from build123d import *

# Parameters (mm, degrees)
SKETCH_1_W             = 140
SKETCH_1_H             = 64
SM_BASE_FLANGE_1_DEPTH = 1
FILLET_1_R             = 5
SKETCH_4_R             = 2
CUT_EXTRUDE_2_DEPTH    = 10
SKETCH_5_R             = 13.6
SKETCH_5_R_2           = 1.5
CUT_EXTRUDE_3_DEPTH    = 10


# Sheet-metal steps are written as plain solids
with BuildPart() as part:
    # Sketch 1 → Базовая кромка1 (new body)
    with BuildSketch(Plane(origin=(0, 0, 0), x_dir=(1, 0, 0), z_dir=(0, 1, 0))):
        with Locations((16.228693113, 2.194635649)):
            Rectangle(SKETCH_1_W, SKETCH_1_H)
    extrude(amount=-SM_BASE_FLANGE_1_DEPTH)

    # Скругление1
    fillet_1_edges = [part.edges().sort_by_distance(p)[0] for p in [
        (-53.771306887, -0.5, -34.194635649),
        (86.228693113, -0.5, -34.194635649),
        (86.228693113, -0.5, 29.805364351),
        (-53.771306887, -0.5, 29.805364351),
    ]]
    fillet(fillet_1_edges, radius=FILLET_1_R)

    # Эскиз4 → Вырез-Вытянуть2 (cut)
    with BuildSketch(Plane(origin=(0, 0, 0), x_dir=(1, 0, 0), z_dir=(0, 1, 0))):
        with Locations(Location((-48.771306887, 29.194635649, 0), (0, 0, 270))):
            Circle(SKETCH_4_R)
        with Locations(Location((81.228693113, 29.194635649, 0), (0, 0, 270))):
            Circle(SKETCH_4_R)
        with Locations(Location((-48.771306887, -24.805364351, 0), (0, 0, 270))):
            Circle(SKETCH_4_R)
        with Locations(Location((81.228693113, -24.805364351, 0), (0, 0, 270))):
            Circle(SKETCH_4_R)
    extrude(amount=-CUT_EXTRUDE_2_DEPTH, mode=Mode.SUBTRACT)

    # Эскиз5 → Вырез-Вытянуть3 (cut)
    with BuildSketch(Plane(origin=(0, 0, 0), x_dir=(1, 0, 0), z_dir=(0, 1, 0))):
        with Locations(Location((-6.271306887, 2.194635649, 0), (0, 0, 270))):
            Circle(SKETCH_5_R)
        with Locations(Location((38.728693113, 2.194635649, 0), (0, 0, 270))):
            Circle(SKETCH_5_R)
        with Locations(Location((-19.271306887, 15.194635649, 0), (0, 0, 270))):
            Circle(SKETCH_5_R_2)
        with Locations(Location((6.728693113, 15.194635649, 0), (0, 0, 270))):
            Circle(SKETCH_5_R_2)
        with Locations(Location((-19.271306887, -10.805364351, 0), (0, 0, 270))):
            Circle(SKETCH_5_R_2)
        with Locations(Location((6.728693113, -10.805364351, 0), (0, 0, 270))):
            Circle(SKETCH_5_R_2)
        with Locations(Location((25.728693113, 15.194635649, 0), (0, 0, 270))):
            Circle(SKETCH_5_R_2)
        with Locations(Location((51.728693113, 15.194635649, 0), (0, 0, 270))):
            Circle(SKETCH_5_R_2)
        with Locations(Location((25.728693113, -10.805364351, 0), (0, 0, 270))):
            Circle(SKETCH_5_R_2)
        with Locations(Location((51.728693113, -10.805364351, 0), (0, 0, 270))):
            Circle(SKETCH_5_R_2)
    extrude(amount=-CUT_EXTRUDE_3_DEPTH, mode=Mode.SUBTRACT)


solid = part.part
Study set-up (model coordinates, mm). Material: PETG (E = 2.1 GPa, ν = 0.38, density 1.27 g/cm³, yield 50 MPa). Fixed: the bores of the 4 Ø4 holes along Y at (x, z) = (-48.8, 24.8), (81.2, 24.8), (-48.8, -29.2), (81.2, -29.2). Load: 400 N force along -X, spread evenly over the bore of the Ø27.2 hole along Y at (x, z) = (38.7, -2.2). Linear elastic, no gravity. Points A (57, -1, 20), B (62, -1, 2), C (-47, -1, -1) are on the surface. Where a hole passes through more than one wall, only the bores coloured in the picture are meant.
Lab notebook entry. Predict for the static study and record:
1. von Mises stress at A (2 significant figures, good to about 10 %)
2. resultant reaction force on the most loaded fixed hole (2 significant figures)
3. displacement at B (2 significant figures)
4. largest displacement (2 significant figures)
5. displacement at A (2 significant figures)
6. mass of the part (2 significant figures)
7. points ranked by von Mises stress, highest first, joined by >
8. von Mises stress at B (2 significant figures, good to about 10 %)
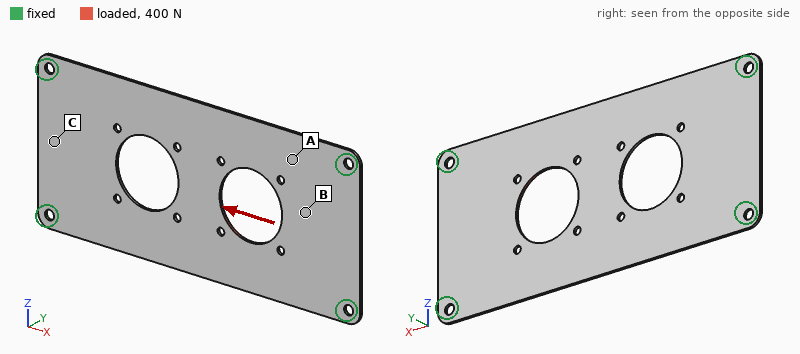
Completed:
5.4 MPa
140 N
0.12 mm
0.19 mm
0.093 mm
9.7 g
A > B > C
3.2 MPa
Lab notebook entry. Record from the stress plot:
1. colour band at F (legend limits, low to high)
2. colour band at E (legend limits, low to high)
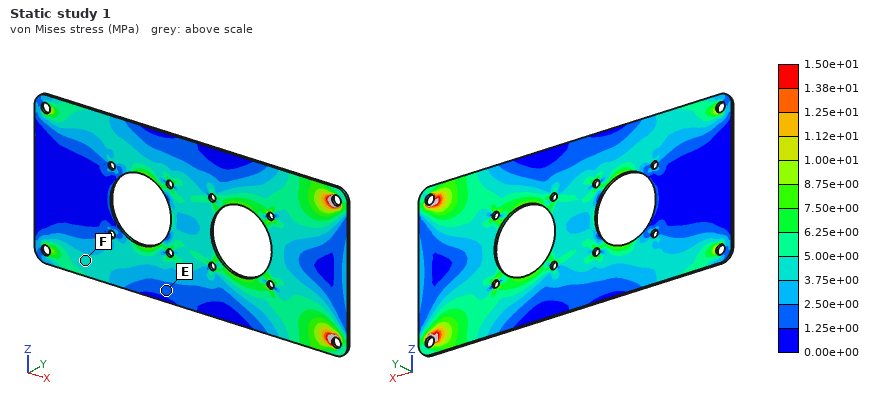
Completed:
3.75e+00 to 5.00e+00 MPa
1.25e+00 to 2.50e+00 MPa
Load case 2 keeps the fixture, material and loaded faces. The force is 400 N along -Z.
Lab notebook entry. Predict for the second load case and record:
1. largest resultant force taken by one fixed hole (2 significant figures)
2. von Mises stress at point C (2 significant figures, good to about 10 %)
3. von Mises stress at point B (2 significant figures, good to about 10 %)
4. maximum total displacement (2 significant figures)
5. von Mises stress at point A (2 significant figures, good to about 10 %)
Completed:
190 N
2.1 MPa
13 MPa
0.52 mm
5.6 MPa
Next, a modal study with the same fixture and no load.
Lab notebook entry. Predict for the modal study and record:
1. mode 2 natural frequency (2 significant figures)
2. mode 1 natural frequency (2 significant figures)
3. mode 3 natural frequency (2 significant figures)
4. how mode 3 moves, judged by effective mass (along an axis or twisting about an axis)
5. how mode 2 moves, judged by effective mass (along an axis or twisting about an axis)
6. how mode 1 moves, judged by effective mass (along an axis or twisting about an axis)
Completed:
130 Hz
76 Hz
200 Hz
twisting about Z
twisting about X
along Y
